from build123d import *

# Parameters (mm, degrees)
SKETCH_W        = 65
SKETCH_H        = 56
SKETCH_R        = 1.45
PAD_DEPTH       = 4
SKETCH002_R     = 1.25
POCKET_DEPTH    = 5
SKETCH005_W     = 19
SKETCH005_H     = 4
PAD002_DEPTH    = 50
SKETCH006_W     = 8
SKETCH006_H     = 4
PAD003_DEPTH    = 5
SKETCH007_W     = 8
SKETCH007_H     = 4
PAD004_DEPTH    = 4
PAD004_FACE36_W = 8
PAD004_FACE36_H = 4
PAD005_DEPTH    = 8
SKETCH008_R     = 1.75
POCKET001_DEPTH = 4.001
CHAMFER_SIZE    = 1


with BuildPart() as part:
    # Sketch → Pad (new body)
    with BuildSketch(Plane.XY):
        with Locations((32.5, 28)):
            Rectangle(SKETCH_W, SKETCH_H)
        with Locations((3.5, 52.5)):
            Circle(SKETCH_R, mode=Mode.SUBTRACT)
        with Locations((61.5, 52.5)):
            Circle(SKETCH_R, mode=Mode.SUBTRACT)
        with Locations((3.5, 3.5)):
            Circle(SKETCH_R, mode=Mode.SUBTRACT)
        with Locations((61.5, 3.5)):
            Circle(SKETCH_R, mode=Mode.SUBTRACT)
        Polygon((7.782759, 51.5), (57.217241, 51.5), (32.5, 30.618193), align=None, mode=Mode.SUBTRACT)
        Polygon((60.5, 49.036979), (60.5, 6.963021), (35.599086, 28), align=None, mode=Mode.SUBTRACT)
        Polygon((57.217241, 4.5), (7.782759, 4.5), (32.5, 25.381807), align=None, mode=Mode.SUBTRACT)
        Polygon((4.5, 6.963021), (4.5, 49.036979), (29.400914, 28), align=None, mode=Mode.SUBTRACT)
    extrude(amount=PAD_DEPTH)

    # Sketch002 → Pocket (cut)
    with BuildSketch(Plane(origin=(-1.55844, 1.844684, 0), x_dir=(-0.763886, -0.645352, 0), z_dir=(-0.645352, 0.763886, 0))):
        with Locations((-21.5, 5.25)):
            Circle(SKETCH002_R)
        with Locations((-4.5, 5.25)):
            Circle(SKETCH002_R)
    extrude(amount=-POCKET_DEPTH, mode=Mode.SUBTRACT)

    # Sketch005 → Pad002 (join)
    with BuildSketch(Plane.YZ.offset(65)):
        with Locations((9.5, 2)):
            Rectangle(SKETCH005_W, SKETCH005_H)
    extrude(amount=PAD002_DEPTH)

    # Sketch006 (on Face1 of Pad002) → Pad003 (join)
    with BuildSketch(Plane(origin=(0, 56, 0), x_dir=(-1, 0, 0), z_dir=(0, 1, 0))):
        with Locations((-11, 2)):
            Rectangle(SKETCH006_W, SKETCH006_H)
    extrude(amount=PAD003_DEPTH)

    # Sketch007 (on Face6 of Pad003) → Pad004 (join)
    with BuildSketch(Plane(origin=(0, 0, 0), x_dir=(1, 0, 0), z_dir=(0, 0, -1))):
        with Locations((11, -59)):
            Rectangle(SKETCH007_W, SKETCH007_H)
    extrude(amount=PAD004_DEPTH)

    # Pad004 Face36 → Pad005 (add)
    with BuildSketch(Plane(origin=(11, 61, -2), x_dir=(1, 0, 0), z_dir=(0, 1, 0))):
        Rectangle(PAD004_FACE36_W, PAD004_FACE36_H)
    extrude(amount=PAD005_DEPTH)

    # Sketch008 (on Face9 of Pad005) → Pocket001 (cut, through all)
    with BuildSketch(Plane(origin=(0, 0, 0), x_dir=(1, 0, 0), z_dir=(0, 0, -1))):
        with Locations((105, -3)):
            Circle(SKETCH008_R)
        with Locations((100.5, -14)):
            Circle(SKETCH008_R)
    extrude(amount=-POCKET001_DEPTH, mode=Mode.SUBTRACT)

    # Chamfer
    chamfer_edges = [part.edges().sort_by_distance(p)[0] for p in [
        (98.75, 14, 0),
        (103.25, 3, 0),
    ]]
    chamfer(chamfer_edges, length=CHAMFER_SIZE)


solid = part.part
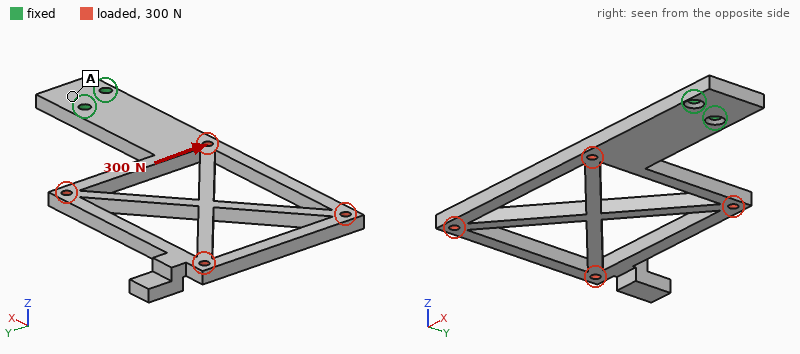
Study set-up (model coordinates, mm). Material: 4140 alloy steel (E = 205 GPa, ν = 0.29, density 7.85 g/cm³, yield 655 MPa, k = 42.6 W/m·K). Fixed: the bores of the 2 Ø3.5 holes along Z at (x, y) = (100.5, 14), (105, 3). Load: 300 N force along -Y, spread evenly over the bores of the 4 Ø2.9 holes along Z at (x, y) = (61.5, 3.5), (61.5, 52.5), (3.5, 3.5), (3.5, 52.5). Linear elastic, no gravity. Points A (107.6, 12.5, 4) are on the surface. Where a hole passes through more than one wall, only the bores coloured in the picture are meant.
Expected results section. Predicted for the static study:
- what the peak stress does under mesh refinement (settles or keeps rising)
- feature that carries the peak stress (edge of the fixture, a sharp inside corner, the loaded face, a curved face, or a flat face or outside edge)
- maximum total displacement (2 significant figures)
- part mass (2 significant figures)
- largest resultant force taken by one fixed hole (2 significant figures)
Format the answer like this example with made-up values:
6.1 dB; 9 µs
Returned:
keeps rising; edge of the fixture; 0.44 mm; 82 g; 1.6 kN
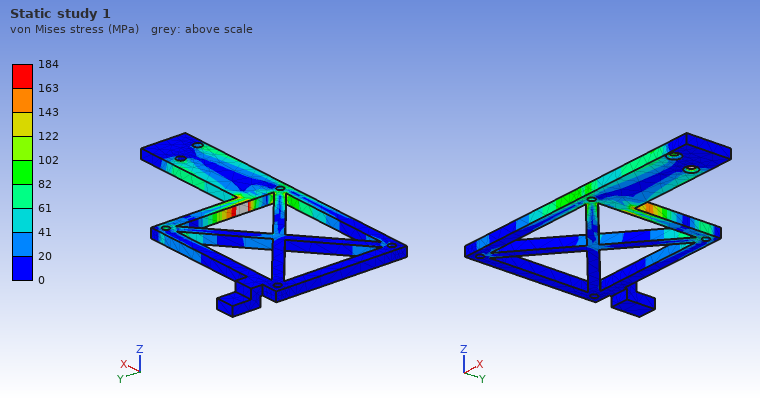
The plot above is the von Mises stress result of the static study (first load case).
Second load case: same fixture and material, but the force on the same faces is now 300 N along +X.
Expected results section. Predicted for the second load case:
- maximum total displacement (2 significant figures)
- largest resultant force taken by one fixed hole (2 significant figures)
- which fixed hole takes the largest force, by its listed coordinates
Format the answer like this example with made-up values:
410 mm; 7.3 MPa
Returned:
0.30 mm; 600 N; (100.5, 14)
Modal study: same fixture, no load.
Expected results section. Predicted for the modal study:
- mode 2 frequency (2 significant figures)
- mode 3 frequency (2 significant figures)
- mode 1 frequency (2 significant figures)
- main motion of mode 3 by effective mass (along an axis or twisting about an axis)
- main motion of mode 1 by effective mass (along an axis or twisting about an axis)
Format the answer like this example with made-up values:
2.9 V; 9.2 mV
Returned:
590 Hz; 620 Hz; 220 Hz; twisting about X; along Z
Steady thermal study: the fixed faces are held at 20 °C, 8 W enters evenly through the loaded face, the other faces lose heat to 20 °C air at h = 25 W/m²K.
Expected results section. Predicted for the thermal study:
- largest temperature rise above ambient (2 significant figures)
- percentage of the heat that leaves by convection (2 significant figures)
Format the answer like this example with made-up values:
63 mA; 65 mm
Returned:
55 K; 78 %
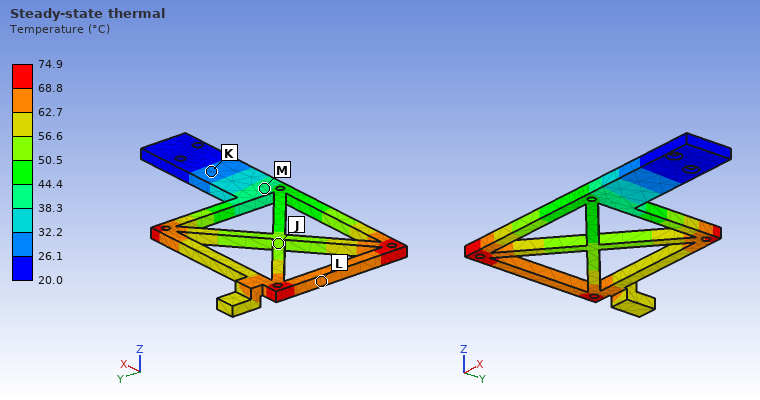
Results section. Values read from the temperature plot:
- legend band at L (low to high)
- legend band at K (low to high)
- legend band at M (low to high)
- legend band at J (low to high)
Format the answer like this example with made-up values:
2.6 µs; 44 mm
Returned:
62.7 to 68.8 °C; 26.1 to 32.2 °C; 38.3 to 44.4 °C; 50.5 to 56.6 °C
